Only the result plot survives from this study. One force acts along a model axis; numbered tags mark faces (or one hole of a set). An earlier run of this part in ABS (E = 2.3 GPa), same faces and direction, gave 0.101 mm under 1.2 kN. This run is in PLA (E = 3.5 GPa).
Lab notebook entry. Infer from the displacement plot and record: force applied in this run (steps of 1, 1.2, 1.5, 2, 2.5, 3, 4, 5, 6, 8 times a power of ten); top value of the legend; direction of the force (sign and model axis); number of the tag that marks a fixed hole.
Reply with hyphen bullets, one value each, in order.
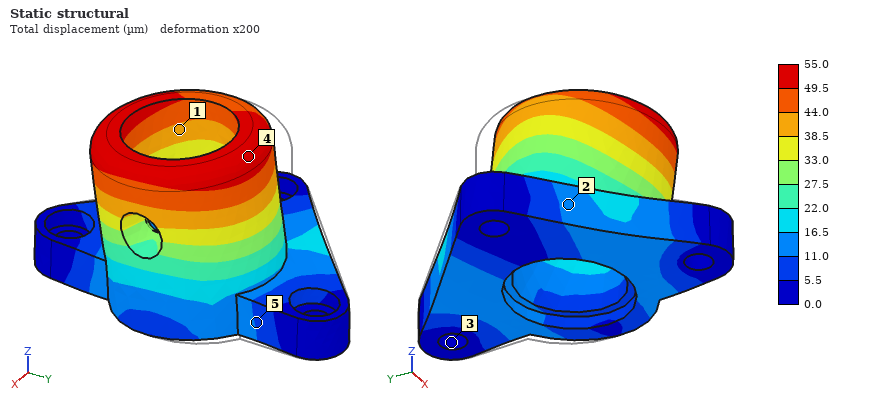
- 1 kN
- 55.0 µm
- -Y
- 3
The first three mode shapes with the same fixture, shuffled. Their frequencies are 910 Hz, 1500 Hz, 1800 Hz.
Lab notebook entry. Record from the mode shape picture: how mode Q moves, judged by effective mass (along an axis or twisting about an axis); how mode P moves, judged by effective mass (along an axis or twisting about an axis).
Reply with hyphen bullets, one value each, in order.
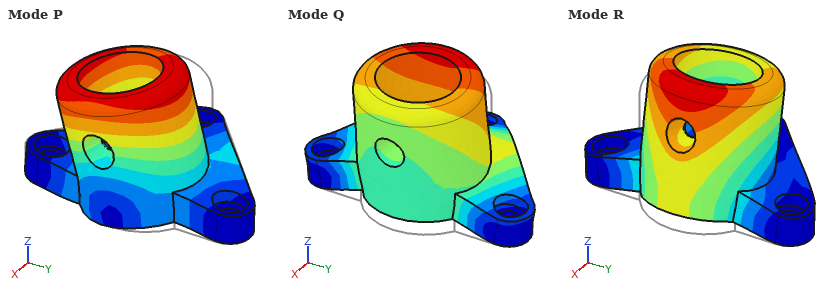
- along Z
- along Y
